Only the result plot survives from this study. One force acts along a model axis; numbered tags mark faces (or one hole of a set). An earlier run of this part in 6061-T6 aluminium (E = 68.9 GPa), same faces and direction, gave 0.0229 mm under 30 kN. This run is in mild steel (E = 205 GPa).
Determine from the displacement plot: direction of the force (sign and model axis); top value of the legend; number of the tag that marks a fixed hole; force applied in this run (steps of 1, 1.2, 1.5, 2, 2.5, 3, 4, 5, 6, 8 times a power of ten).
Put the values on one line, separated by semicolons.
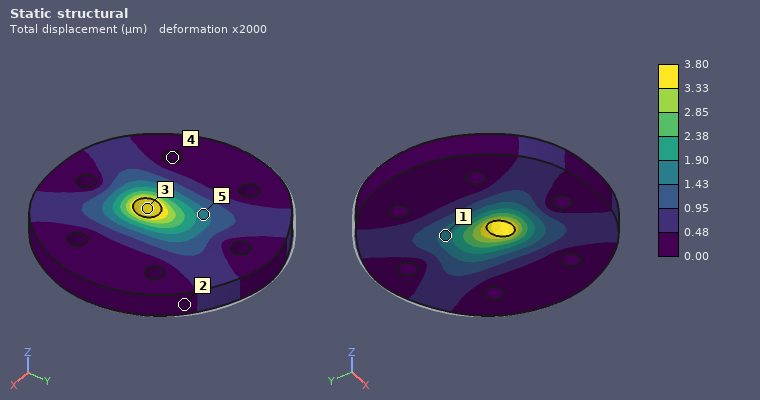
-Y; 3.80 µm; 4; 15 kN
